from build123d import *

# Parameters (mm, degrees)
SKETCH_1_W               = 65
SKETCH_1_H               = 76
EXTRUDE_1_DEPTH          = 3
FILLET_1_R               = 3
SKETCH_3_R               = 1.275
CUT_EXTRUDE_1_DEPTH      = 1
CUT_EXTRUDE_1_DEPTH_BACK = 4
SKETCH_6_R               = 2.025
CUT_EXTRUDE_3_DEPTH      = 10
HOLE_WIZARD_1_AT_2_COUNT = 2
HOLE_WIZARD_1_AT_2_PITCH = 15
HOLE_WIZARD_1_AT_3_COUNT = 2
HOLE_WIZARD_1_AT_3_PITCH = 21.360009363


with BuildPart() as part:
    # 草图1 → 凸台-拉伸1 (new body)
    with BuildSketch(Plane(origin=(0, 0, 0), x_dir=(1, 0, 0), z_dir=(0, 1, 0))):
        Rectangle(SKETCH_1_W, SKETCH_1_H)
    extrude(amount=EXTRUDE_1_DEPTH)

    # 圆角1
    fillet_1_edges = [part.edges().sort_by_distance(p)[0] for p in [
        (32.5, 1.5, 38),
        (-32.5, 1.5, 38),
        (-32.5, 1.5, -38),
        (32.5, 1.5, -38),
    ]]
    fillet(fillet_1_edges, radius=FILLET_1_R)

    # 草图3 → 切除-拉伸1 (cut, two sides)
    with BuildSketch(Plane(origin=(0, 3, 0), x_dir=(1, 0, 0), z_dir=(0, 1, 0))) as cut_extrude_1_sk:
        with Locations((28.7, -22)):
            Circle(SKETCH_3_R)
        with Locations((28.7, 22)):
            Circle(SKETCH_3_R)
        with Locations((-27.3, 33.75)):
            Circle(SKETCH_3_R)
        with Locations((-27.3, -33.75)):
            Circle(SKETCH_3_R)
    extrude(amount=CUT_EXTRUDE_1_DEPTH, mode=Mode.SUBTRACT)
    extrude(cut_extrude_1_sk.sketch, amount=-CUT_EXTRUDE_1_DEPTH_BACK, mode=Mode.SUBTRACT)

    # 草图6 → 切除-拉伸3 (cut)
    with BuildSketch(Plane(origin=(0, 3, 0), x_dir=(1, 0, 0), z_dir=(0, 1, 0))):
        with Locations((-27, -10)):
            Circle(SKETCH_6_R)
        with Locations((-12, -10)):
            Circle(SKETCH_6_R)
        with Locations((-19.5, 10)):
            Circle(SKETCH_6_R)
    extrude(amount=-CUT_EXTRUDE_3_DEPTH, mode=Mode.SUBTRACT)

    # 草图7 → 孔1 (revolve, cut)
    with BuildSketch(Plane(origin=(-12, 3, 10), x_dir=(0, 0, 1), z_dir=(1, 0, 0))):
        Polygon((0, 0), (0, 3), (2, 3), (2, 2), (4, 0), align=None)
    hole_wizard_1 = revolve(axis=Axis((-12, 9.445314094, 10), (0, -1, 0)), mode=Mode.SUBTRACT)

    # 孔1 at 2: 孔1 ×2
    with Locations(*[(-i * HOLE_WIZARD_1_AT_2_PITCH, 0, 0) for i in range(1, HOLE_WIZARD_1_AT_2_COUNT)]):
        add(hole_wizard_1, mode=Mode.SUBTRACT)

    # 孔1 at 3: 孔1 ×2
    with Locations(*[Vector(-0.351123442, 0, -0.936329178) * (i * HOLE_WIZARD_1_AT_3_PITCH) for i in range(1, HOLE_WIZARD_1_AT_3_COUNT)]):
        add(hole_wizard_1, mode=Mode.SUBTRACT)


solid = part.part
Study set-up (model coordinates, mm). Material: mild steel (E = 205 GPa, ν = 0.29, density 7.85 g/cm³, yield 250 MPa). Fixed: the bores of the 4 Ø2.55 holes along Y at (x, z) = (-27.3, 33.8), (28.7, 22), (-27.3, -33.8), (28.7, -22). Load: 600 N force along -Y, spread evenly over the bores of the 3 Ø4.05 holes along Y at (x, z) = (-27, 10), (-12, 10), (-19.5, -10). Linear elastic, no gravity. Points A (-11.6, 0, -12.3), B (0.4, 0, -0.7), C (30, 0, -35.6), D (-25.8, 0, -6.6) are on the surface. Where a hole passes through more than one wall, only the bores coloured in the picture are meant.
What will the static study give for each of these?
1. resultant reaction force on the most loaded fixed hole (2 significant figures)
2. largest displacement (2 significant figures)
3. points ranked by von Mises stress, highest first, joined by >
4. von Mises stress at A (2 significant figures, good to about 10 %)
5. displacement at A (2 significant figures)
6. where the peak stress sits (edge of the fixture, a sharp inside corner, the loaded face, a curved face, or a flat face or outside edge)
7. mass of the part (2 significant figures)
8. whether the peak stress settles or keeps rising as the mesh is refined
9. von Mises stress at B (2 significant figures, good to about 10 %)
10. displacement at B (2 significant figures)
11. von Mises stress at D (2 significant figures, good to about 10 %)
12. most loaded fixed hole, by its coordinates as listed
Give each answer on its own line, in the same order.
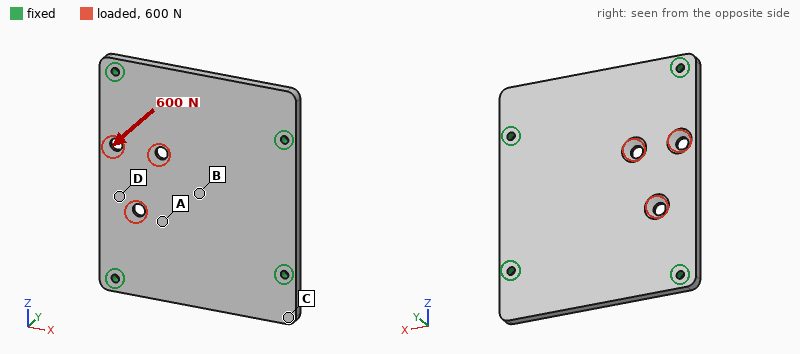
300 N
76 µm
D > A > B > C
40 MPa
44 µm
edge of the fixture
110 g
keeps rising
26 MPa
39 µm
59 MPa
(-27.3, 33.8)
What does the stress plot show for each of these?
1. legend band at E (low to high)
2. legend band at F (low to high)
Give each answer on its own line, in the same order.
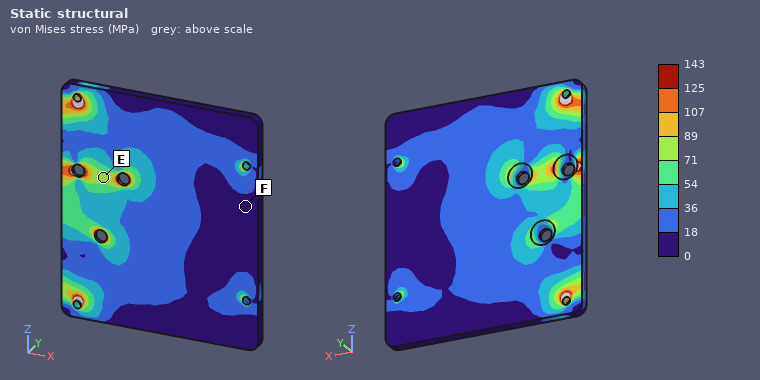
71 to 89 MPa
0 to 18 MPa
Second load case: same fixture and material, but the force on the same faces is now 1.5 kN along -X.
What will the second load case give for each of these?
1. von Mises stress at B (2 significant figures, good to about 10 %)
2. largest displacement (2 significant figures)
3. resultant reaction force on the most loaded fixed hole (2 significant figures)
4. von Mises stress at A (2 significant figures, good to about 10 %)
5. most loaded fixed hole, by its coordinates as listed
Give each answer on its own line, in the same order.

13 MPa
9.9 µm
470 N
17 MPa
(28.7, 22)
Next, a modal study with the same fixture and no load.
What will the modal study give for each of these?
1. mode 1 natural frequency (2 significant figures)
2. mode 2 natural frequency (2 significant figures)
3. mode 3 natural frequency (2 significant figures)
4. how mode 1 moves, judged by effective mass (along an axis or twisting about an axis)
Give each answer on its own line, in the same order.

2900 Hz
4500 Hz
4500 Hz
along Y
